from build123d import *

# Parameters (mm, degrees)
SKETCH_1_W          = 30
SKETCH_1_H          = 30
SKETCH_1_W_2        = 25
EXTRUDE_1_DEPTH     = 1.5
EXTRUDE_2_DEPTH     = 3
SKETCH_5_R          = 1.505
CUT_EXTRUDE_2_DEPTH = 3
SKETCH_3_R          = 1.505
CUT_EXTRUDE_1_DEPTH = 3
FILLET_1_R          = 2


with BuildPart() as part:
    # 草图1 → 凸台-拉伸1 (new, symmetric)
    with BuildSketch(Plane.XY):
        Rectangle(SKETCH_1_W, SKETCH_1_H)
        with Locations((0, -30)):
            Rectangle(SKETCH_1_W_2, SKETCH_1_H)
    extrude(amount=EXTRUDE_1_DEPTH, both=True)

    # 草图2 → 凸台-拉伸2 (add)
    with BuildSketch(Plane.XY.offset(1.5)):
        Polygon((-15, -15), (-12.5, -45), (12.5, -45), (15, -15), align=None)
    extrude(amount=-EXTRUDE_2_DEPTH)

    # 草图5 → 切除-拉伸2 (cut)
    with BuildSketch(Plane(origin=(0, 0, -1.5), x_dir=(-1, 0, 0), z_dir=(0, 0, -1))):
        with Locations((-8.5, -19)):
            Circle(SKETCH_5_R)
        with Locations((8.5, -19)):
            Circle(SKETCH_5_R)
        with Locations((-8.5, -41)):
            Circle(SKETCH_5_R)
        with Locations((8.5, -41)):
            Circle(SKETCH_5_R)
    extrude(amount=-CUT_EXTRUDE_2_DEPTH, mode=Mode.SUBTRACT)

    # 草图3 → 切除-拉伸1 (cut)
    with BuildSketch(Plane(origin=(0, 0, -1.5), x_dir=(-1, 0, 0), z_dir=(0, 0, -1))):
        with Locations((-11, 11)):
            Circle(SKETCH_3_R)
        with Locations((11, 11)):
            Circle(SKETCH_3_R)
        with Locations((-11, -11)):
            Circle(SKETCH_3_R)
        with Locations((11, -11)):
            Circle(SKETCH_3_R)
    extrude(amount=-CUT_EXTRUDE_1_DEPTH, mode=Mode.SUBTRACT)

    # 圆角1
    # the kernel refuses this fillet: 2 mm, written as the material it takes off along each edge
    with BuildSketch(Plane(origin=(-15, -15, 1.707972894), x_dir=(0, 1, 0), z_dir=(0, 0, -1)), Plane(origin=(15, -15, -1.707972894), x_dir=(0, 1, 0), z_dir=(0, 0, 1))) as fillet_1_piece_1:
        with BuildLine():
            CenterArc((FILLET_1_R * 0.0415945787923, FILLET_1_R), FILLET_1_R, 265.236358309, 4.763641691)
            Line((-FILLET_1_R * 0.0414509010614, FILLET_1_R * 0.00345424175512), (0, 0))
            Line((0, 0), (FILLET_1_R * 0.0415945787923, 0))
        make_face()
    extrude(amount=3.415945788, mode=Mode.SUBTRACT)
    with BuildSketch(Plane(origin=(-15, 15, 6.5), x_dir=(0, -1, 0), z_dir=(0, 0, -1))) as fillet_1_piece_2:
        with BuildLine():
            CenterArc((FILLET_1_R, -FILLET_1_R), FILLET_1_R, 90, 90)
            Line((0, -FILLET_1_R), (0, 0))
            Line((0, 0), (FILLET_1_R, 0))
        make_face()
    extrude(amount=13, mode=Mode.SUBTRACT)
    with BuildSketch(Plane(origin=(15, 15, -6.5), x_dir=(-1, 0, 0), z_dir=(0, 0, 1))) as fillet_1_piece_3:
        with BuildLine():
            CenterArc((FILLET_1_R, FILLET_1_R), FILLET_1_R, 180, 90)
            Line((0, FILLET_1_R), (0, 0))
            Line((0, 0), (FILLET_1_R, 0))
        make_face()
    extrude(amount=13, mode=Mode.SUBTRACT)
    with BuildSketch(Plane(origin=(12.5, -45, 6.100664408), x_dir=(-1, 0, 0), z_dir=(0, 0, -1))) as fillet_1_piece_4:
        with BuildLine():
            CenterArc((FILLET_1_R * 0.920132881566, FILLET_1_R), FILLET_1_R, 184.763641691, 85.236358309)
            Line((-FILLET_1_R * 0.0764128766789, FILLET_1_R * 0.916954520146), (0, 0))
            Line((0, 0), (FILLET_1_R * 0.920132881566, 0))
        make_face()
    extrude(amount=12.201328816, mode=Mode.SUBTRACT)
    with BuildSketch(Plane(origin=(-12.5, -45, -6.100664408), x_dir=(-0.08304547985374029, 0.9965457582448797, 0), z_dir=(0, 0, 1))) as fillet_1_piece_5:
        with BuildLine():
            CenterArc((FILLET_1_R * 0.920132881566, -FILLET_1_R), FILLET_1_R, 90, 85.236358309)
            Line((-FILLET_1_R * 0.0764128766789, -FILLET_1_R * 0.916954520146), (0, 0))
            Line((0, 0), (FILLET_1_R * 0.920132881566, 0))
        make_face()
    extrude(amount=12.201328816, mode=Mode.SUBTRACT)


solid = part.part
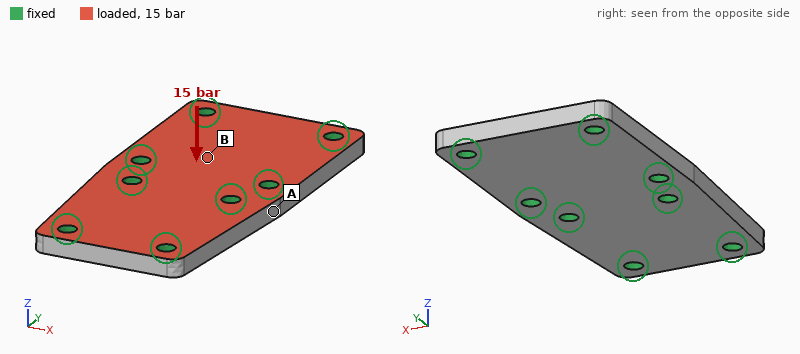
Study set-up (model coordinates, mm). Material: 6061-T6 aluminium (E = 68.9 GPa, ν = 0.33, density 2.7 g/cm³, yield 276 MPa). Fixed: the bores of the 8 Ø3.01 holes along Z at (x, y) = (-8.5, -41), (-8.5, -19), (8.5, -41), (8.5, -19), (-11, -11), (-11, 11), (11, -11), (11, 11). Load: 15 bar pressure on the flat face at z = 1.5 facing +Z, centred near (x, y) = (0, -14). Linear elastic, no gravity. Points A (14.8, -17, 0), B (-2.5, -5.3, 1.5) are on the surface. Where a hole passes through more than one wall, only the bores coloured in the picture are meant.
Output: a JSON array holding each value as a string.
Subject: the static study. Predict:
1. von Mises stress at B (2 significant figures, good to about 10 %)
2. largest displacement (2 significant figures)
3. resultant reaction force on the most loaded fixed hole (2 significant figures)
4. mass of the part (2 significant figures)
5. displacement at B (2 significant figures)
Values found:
["15 MPa", "13 µm", "340 N", "13 g", "10 µm"]
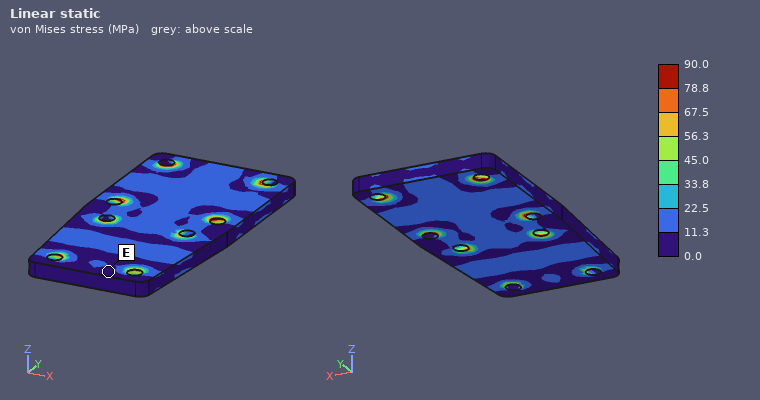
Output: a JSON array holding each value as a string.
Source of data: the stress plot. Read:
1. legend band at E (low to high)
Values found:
["0.0 to 11.3 MPa"]
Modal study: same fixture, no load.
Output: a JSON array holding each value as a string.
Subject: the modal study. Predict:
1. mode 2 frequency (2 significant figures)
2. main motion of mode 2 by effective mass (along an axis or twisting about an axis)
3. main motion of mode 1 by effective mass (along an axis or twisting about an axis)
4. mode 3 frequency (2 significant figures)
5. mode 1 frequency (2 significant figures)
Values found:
["28 kHz", "along Z", "along Z", "33 kHz", "23 kHz"]
